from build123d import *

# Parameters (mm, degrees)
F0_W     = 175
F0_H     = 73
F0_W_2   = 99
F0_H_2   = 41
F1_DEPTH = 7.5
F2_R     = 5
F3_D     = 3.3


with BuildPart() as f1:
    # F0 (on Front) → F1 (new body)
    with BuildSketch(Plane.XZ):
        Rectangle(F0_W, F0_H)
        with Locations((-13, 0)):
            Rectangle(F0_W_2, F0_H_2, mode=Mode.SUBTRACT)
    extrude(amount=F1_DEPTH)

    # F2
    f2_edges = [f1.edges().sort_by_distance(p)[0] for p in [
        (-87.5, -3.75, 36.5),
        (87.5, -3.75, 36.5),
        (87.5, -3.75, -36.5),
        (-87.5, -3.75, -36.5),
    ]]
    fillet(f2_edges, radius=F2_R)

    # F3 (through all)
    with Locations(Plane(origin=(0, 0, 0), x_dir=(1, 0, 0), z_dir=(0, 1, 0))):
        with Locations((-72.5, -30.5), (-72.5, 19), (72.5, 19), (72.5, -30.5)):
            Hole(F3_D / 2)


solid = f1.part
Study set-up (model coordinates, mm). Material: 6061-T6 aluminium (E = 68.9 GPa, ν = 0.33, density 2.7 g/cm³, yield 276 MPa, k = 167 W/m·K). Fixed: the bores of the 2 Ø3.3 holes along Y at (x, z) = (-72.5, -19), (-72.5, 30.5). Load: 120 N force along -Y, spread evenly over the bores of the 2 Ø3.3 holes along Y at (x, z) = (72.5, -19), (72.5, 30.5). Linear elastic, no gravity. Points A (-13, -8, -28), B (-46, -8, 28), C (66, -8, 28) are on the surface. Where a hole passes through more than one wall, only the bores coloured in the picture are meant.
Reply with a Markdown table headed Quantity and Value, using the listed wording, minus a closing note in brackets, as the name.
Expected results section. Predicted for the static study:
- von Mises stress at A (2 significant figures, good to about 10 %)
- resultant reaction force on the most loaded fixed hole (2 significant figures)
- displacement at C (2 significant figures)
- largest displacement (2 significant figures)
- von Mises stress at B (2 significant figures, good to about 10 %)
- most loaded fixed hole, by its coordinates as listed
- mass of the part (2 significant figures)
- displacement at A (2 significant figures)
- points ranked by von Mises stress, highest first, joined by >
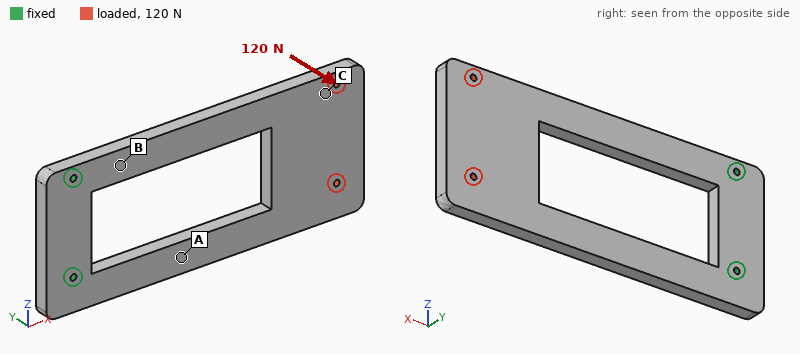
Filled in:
| Quantity | Value |
|---|---|
| von Mises stress at A | 34 MPa |
| resultant reaction force on the most loaded fixed hole | 86 N |
| displacement at C | 1.5 mm |
| largest displacement | 1.8 mm |
| von Mises stress at B | 49 MPa |
| most loaded fixed hole, by its coordinates as listed | (-72.5, 30.5) |
| mass of the part | 180 g |
| displacement at A | 0.35 mm |
| points ranked by von Mises stress, highest first, joined by > | B > A > C |
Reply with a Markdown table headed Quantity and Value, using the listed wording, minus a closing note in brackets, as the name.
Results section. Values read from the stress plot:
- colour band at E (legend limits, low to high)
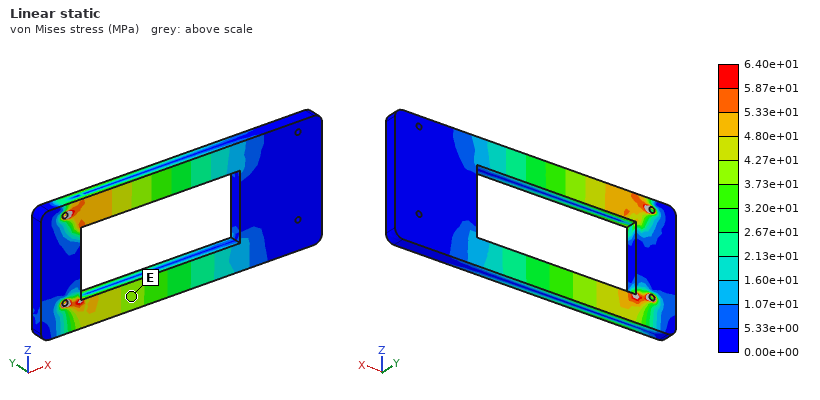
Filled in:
| Quantity | Value |
|---|---|
| colour band at E | 3.73e+01 to 4.27e+01 MPa |
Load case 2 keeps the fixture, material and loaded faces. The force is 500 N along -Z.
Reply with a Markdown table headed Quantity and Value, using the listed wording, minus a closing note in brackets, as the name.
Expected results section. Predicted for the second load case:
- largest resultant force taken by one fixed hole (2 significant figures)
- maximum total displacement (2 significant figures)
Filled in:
| Quantity | Value |
|---|---|
| largest resultant force taken by one fixed hole | 1.5 kN |
| maximum total displacement | 0.26 mm |
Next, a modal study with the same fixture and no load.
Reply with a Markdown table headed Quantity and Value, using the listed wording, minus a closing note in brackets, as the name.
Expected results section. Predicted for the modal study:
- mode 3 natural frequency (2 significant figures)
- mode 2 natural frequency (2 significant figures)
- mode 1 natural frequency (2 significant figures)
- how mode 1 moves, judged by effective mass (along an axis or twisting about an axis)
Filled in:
| Quantity | Value |
|---|---|
| mode 3 natural frequency | 740 Hz |
| mode 2 natural frequency | 720 Hz |
| mode 1 natural frequency | 170 Hz |
| how mode 1 moves, judged by effective mass | along Y |
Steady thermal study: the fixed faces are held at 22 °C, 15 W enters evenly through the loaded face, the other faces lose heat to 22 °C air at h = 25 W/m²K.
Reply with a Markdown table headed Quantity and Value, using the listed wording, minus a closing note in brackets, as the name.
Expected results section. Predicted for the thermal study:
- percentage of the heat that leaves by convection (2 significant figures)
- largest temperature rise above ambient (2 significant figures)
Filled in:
| Quantity | Value |
|---|---|
| percentage of the heat that leaves by convection | 55 % |
| largest temperature rise above ambient | 29 K |
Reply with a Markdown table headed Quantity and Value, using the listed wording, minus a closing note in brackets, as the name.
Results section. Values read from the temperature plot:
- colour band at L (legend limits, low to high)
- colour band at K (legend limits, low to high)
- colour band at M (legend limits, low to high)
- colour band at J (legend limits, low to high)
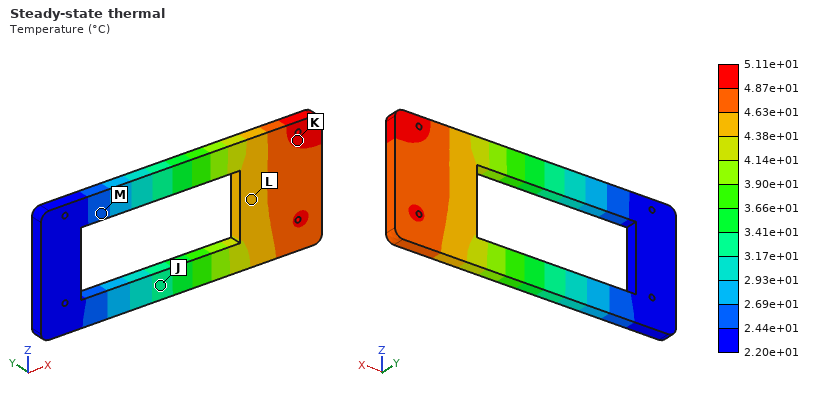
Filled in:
| Quantity | Value |
|---|---|
| colour band at L | 4.38e+01 to 4.63e+01 °C |
| colour band at K | 4.87e+01 to 5.11e+01 °C |
| colour band at M | 2.44e+01 to 2.69e+01 °C |
| colour band at J | 3.17e+01 to 3.41e+01 °C |
